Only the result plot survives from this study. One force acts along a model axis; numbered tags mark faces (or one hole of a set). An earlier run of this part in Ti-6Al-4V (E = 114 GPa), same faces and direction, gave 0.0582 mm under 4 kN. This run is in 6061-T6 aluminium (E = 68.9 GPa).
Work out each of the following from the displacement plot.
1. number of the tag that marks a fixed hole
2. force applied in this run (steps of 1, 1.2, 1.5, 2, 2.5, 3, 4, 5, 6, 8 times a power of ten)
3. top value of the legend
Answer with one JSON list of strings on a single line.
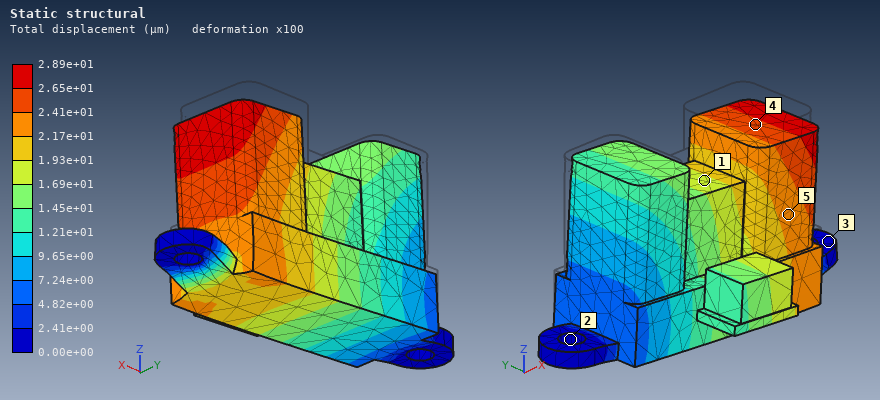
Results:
["2", "1.2 kN", "2.89e+01 µm"]
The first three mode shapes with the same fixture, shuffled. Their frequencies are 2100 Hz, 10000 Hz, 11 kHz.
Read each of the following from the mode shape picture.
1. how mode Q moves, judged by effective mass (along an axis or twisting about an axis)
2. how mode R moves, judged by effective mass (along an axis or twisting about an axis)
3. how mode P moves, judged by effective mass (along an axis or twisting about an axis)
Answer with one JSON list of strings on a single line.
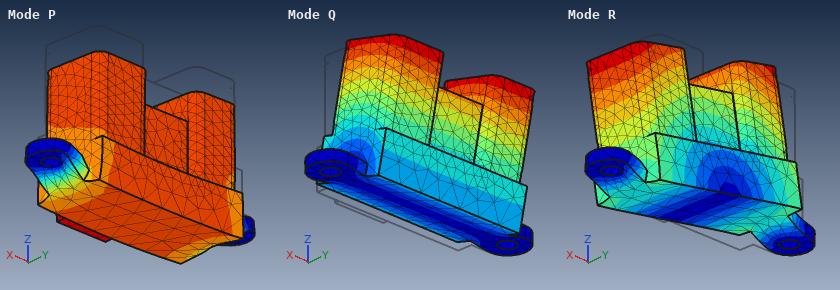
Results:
["along Y", "along X", "along Z"]
